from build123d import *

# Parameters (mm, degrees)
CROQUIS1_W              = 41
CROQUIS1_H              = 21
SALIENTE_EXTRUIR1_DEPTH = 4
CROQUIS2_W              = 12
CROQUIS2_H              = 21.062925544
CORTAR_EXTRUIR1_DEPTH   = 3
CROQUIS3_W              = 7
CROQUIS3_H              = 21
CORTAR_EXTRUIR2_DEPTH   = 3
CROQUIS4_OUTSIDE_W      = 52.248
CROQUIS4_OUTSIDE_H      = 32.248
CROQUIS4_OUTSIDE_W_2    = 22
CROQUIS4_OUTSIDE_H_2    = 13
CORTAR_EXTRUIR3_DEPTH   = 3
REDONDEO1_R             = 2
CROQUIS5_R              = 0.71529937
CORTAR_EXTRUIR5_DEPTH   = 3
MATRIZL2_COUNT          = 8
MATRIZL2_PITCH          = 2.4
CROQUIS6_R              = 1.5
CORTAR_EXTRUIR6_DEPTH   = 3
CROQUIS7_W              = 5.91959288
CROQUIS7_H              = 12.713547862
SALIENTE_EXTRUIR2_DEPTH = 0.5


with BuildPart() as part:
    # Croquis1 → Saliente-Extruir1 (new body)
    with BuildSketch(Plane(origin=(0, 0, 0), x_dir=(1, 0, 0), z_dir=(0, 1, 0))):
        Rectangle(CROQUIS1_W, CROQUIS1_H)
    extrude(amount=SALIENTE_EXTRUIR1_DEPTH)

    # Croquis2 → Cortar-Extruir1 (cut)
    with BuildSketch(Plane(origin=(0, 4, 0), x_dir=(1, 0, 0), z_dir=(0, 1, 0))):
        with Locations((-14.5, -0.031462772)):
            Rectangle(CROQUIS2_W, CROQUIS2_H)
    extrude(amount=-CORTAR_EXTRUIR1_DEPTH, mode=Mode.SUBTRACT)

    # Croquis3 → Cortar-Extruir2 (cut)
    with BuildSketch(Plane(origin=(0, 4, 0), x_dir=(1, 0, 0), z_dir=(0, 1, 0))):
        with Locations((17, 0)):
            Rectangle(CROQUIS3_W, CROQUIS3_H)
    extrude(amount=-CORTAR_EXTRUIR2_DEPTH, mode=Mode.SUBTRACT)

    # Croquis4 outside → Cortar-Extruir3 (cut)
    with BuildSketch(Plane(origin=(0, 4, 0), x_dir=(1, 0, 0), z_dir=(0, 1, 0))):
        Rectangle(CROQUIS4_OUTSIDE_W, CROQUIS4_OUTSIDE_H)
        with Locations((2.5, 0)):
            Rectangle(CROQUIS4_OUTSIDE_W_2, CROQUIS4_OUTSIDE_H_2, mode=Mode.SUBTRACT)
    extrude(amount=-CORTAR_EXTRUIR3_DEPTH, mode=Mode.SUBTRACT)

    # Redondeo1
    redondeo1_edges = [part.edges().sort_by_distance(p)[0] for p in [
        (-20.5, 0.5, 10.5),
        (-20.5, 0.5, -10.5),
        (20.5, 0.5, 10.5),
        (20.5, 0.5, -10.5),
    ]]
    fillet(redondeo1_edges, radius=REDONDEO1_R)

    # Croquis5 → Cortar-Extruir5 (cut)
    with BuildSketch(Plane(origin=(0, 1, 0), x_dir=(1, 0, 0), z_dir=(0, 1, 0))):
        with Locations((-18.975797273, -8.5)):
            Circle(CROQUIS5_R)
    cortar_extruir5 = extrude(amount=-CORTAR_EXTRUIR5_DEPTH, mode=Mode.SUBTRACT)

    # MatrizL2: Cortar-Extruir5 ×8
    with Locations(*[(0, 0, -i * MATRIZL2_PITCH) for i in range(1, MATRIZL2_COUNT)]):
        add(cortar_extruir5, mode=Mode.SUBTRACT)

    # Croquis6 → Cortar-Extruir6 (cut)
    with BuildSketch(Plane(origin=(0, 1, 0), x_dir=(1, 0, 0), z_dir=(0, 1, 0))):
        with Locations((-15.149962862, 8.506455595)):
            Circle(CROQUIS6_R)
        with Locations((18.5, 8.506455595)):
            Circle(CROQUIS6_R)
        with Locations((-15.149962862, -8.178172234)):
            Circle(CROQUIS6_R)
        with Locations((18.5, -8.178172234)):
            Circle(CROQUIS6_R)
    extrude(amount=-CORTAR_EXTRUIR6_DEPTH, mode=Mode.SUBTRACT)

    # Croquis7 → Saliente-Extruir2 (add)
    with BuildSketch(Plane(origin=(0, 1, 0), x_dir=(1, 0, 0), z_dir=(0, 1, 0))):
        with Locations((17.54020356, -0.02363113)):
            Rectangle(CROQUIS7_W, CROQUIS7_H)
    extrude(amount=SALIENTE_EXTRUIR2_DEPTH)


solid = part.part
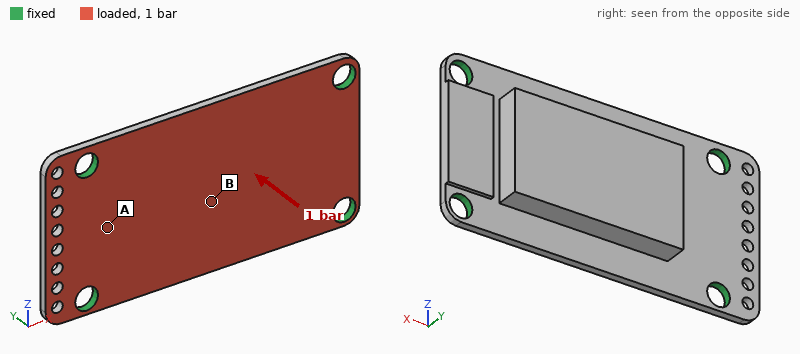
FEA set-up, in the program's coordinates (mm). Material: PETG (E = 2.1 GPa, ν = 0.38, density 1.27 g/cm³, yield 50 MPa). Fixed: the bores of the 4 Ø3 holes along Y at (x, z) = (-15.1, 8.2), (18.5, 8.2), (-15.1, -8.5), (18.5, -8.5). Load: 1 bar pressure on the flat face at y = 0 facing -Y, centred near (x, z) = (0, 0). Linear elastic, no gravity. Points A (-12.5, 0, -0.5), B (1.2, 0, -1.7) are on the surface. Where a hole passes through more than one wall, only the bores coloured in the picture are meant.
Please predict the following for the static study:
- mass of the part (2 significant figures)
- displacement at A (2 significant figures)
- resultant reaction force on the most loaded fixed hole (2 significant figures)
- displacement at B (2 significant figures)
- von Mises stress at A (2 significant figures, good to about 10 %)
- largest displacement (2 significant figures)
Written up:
2.2 g
0.18 mm
27 N
0.26 mm
6.7 MPa
0.31 mm
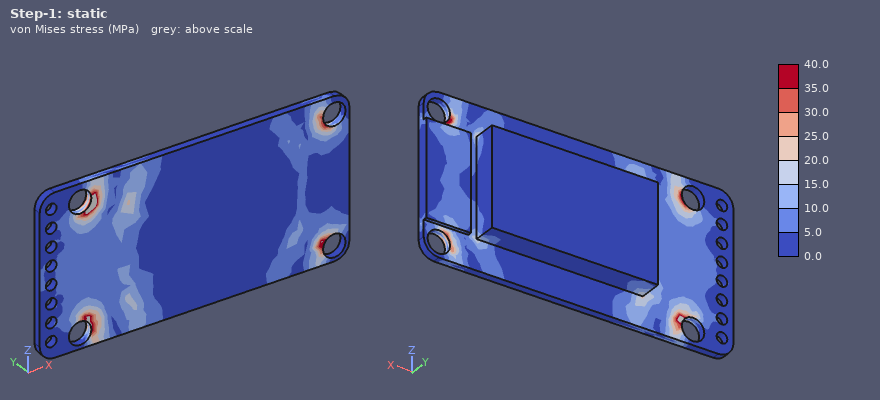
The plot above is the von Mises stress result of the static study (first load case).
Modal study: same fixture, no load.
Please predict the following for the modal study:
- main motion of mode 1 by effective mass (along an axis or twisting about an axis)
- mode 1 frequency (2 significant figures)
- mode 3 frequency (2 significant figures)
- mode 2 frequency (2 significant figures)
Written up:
along Y
1800 Hz
4000 Hz
2800 Hz
